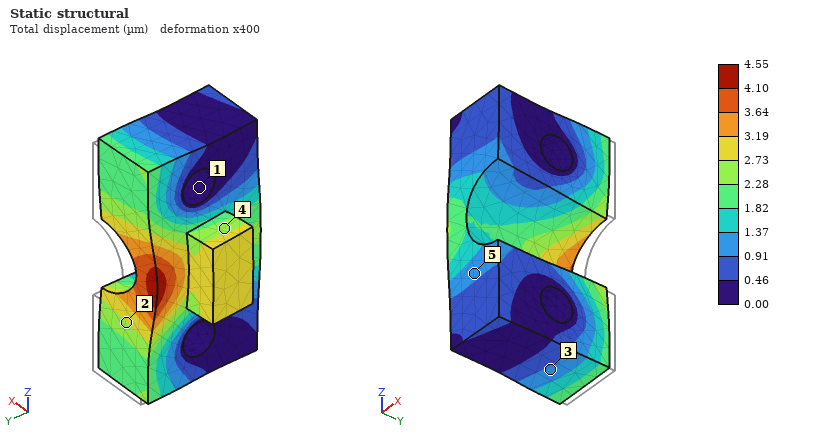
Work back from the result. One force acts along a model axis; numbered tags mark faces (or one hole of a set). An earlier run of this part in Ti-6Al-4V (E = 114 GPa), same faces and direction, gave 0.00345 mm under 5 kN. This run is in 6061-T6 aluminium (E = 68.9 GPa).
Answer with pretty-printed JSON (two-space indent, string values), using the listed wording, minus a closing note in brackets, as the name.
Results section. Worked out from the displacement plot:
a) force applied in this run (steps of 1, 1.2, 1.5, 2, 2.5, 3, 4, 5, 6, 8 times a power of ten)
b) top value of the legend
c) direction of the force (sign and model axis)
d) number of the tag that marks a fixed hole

{
  "force applied in this run": "4 kN",
  "top value of the legend": "4.55 µm",
  "direction of the force": "-Y",
  "number of the tag that marks a fixed hole": "1"
}
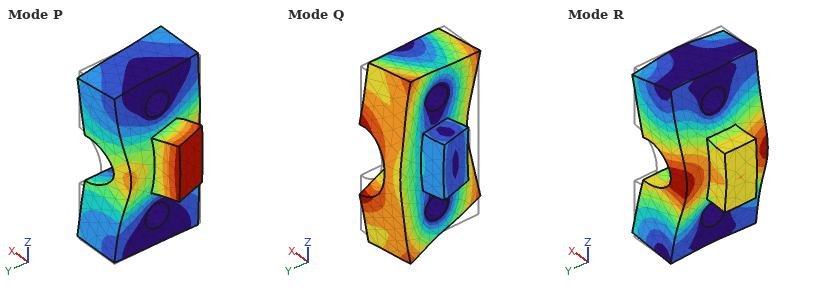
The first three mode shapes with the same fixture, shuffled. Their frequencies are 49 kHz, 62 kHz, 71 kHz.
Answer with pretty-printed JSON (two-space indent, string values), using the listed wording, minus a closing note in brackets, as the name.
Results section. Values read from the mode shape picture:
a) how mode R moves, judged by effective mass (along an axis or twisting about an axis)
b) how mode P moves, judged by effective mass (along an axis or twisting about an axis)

{
  "how mode R moves, judged by effective mass": "along X",
  "how mode P moves, judged by effective mass": "along Y"
}
